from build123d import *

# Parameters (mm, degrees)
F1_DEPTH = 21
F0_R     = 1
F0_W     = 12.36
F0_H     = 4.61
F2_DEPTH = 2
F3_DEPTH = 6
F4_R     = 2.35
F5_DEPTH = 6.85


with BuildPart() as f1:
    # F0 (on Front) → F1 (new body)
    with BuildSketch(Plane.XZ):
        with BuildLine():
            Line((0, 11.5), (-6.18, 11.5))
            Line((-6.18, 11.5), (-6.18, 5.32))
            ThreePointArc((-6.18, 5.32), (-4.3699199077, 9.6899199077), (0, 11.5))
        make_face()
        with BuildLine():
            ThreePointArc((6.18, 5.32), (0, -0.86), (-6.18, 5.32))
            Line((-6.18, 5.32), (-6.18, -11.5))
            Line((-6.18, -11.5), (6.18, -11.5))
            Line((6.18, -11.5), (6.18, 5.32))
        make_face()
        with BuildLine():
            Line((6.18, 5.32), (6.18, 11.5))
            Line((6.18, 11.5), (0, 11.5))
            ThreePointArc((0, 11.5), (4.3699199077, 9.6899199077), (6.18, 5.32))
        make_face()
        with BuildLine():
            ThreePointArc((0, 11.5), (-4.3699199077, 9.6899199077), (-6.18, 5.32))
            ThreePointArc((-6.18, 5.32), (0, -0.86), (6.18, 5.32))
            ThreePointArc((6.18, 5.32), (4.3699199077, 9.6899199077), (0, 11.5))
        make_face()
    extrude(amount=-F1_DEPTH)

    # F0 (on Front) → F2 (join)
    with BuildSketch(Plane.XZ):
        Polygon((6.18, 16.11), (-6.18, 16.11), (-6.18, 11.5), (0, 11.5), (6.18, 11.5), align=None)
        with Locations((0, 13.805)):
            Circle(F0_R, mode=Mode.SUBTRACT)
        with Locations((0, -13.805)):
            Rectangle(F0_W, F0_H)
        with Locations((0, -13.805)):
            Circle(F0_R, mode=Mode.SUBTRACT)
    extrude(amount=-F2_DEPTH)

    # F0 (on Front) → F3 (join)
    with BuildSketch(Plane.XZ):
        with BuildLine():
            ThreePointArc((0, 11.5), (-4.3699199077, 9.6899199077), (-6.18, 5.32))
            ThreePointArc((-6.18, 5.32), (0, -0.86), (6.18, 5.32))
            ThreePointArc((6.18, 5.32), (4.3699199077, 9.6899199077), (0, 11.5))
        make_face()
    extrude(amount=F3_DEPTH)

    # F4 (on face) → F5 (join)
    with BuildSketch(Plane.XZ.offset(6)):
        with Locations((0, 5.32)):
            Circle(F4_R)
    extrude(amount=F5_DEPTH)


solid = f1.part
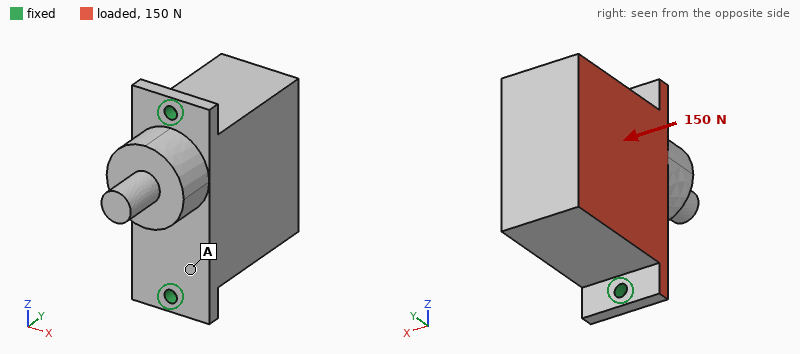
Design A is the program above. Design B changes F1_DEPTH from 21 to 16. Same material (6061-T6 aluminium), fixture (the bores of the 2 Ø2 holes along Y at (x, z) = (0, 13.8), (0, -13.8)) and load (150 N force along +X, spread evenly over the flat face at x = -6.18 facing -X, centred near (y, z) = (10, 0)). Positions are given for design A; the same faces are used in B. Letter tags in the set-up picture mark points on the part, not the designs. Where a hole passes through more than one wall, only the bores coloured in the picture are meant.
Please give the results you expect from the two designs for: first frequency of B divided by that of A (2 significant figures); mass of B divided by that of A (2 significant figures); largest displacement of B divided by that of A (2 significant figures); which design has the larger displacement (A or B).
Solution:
1.4
0.80
0.57
A
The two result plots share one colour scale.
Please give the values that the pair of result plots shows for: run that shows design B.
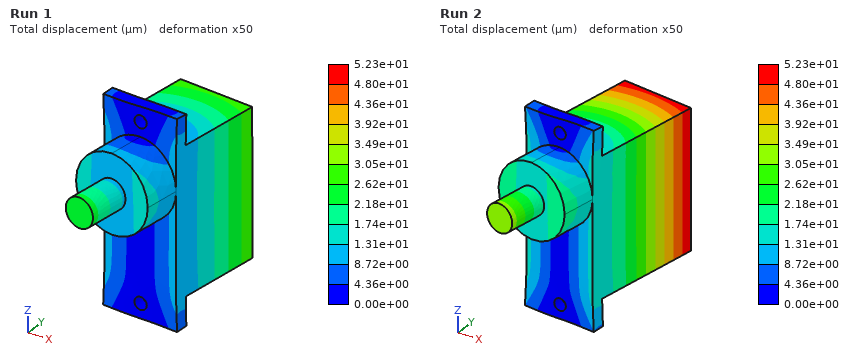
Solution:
Run 1
